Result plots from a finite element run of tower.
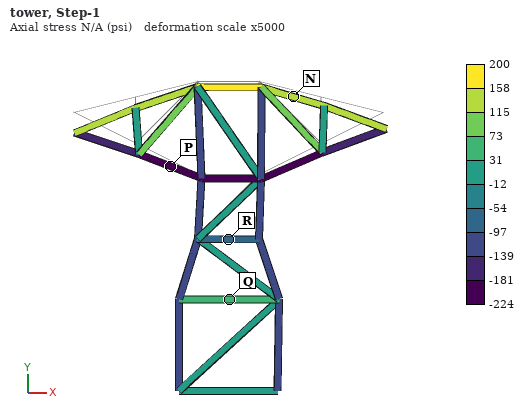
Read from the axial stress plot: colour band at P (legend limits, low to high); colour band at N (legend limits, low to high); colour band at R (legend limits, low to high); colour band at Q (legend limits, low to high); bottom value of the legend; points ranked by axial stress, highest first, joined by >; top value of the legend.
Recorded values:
-224 to -181 psi
115 to 158 psi
-97 to -54 psi
31 to 73 psi
-224 psi
N > Q > R > P
200 psi
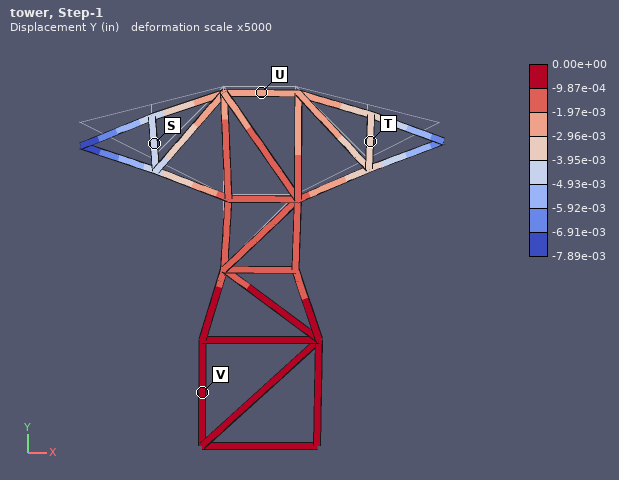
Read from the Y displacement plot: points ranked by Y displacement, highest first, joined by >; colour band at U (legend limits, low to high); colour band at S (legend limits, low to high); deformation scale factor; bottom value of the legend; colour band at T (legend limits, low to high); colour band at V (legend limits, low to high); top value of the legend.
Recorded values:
V > U > T > S
-2.96e-03 to -1.97e-03 in
-4.93e-03 to -3.95e-03 in
5000
-7.89e-03 in
-3.95e-03 to -2.96e-03 in
-9.87e-04 to 0.00e+00 in
0.00e+00 in
